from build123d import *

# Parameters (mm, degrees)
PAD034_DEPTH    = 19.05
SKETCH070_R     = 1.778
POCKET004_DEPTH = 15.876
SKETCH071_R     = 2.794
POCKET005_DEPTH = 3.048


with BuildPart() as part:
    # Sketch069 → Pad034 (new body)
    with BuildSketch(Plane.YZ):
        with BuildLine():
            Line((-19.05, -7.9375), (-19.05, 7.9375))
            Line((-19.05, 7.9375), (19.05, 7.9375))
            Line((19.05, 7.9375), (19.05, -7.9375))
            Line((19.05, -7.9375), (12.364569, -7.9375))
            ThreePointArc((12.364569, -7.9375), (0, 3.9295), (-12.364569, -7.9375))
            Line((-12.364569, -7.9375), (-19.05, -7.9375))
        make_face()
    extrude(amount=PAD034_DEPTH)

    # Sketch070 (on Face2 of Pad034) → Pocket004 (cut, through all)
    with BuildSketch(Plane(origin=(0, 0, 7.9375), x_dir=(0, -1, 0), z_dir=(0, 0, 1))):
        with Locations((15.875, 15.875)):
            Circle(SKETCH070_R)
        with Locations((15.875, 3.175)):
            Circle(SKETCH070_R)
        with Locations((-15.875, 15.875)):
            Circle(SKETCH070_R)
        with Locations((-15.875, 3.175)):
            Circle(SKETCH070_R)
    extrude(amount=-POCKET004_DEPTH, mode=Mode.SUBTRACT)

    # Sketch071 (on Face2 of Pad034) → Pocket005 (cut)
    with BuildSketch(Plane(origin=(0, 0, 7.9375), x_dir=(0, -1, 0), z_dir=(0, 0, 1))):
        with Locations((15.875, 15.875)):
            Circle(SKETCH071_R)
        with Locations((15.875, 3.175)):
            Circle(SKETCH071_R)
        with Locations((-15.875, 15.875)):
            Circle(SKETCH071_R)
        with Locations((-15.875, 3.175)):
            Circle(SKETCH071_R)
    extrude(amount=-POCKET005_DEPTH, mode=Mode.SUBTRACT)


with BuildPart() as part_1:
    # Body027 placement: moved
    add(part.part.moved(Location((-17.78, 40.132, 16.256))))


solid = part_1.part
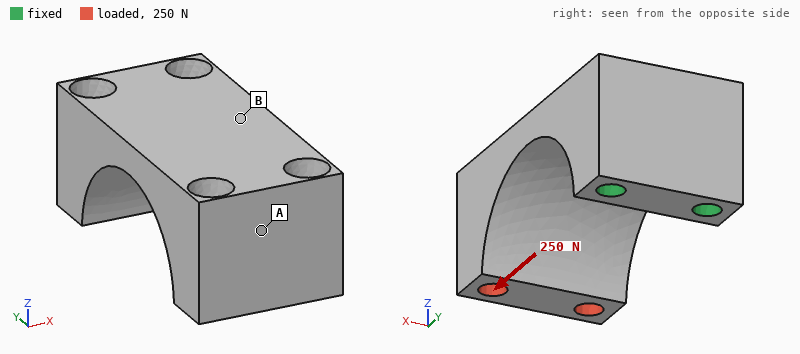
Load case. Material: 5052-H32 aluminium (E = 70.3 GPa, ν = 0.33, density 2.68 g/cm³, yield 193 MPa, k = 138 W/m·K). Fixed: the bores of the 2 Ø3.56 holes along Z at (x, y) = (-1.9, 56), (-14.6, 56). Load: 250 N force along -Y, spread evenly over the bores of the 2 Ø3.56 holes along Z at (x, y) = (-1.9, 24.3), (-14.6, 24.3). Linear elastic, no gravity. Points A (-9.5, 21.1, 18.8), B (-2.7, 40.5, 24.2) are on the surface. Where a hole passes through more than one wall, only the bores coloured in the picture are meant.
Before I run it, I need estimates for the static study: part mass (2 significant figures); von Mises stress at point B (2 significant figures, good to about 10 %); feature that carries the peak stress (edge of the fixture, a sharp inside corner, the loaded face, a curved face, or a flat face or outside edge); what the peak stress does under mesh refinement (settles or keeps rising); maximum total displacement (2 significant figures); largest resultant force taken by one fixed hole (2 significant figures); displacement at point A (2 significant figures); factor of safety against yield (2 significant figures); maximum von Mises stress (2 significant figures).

17 g
29 MPa
a curved face
settles
69 µm
130 N
56 µm
5.0
39 MPa
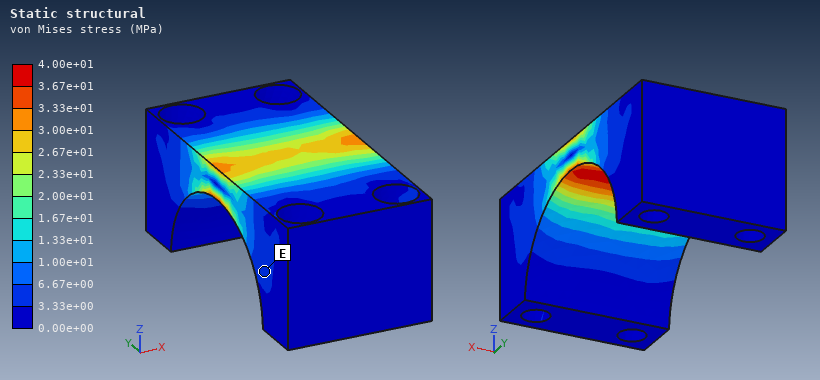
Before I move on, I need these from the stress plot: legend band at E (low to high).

3.33e+00 to 6.67e+00 MPa
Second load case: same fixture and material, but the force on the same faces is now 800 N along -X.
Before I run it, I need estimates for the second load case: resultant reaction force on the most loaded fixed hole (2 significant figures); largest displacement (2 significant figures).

1.8 kN
0.15 mm
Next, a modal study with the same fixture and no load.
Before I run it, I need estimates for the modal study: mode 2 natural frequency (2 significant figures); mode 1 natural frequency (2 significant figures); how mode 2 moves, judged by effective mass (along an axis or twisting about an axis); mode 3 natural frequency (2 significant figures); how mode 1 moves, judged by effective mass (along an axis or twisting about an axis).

5900 Hz
2800 Hz
along X
12 kHz
along Z
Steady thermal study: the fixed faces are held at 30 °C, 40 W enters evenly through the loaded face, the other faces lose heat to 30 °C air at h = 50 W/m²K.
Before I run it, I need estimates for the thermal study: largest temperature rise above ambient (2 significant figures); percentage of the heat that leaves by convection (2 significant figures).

80 K
15 %
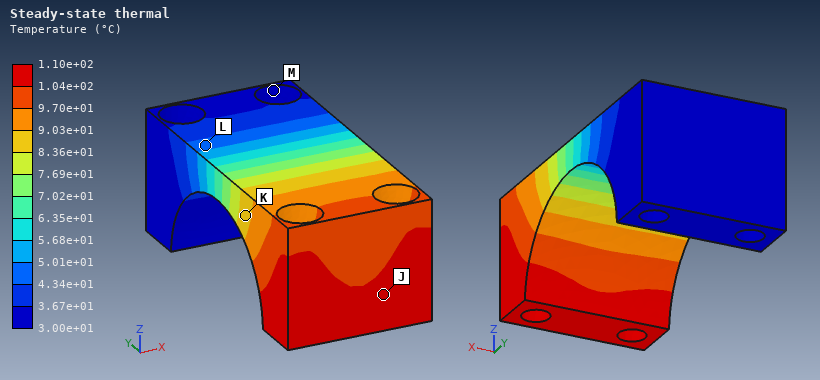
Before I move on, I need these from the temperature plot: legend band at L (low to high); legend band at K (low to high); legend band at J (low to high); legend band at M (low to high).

4.34e+01 to 5.01e+01 °C
8.36e+01 to 9.03e+01 °C
1.04e+02 to 1.10e+02 °C
3.00e+01 to 3.67e+01 °C
